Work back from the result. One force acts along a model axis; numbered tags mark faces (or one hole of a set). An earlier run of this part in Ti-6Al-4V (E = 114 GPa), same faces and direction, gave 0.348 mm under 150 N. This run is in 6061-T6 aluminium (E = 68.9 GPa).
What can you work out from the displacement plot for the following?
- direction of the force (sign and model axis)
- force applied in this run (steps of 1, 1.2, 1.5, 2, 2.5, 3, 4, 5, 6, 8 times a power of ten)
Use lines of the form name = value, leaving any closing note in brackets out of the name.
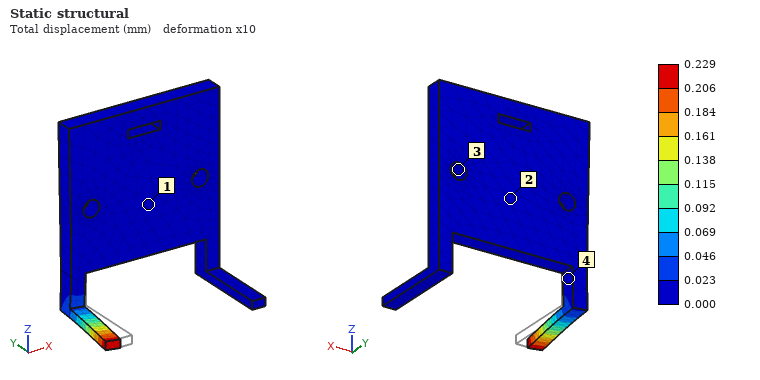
direction of the force = -X
force applied in this run = 60 N
